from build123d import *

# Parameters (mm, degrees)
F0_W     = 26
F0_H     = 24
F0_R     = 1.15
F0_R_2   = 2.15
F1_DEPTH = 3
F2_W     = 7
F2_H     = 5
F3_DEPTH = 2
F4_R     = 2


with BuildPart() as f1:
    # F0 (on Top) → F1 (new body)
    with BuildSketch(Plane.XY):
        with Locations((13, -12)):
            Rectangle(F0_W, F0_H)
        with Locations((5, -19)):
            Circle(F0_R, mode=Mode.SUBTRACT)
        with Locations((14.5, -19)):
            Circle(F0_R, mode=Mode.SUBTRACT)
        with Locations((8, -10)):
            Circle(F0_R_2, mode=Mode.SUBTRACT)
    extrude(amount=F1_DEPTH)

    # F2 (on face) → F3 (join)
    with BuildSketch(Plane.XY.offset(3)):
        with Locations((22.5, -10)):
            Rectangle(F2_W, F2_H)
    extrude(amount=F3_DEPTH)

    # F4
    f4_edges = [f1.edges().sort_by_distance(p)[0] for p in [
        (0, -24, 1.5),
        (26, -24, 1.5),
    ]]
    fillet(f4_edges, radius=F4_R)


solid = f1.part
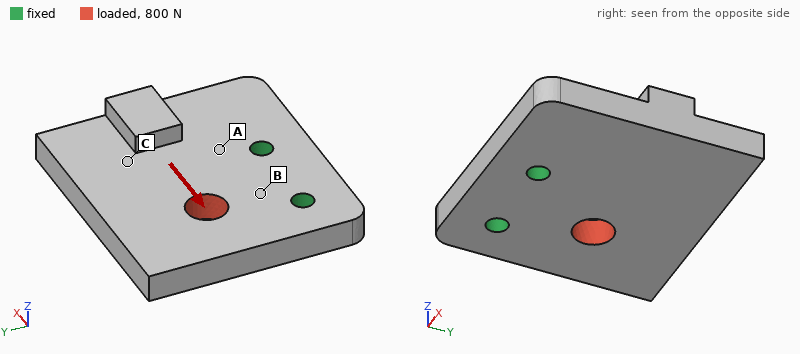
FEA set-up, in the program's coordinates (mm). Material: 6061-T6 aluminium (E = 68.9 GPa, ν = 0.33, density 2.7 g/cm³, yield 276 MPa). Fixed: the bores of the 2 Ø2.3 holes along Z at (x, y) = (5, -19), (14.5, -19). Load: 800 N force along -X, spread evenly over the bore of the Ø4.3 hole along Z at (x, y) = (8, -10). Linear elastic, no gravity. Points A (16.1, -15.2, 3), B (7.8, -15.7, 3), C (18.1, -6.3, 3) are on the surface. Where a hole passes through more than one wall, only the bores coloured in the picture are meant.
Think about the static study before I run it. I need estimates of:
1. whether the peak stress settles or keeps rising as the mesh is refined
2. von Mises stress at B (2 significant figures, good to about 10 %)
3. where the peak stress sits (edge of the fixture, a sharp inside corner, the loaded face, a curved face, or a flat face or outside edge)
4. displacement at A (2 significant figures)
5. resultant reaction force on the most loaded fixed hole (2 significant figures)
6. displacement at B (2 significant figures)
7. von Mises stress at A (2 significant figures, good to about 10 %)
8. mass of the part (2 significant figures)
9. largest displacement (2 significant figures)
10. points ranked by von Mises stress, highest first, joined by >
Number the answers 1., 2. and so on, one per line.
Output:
1. keeps rising
2. 45 MPa
3. edge of the fixture
4. 4.1 µm
5. 740 N
6. 2.7 µm
7. 19 MPa
8. 5.0 g
9. 18 µm
10. B > A > C
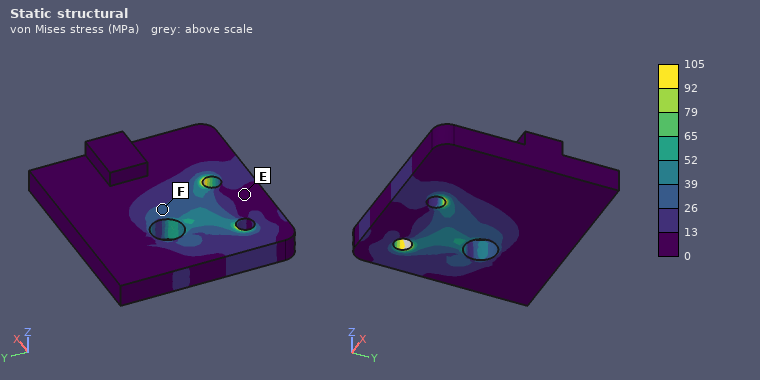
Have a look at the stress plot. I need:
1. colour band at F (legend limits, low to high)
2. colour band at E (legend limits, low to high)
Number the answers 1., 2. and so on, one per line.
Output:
1. 26 to 39 MPa
2. 0 to 13 MPa
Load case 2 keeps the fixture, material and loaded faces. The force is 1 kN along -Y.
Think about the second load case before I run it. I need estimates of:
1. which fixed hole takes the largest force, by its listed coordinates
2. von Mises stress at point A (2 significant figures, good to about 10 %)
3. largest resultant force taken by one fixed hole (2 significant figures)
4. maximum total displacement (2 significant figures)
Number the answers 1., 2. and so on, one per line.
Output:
1. (5, -19)
2. 9.4 MPa
3. 670 N
4. 5.3 µm
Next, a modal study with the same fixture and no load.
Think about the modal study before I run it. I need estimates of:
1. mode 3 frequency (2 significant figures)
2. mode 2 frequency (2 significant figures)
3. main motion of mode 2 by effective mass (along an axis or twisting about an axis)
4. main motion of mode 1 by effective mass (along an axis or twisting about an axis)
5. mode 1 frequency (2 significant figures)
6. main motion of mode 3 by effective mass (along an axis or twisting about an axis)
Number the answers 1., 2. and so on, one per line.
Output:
1. 17 kHz
2. 9900 Hz
3. twisting about Y
4. along Z
5. 5900 Hz
6. along X
